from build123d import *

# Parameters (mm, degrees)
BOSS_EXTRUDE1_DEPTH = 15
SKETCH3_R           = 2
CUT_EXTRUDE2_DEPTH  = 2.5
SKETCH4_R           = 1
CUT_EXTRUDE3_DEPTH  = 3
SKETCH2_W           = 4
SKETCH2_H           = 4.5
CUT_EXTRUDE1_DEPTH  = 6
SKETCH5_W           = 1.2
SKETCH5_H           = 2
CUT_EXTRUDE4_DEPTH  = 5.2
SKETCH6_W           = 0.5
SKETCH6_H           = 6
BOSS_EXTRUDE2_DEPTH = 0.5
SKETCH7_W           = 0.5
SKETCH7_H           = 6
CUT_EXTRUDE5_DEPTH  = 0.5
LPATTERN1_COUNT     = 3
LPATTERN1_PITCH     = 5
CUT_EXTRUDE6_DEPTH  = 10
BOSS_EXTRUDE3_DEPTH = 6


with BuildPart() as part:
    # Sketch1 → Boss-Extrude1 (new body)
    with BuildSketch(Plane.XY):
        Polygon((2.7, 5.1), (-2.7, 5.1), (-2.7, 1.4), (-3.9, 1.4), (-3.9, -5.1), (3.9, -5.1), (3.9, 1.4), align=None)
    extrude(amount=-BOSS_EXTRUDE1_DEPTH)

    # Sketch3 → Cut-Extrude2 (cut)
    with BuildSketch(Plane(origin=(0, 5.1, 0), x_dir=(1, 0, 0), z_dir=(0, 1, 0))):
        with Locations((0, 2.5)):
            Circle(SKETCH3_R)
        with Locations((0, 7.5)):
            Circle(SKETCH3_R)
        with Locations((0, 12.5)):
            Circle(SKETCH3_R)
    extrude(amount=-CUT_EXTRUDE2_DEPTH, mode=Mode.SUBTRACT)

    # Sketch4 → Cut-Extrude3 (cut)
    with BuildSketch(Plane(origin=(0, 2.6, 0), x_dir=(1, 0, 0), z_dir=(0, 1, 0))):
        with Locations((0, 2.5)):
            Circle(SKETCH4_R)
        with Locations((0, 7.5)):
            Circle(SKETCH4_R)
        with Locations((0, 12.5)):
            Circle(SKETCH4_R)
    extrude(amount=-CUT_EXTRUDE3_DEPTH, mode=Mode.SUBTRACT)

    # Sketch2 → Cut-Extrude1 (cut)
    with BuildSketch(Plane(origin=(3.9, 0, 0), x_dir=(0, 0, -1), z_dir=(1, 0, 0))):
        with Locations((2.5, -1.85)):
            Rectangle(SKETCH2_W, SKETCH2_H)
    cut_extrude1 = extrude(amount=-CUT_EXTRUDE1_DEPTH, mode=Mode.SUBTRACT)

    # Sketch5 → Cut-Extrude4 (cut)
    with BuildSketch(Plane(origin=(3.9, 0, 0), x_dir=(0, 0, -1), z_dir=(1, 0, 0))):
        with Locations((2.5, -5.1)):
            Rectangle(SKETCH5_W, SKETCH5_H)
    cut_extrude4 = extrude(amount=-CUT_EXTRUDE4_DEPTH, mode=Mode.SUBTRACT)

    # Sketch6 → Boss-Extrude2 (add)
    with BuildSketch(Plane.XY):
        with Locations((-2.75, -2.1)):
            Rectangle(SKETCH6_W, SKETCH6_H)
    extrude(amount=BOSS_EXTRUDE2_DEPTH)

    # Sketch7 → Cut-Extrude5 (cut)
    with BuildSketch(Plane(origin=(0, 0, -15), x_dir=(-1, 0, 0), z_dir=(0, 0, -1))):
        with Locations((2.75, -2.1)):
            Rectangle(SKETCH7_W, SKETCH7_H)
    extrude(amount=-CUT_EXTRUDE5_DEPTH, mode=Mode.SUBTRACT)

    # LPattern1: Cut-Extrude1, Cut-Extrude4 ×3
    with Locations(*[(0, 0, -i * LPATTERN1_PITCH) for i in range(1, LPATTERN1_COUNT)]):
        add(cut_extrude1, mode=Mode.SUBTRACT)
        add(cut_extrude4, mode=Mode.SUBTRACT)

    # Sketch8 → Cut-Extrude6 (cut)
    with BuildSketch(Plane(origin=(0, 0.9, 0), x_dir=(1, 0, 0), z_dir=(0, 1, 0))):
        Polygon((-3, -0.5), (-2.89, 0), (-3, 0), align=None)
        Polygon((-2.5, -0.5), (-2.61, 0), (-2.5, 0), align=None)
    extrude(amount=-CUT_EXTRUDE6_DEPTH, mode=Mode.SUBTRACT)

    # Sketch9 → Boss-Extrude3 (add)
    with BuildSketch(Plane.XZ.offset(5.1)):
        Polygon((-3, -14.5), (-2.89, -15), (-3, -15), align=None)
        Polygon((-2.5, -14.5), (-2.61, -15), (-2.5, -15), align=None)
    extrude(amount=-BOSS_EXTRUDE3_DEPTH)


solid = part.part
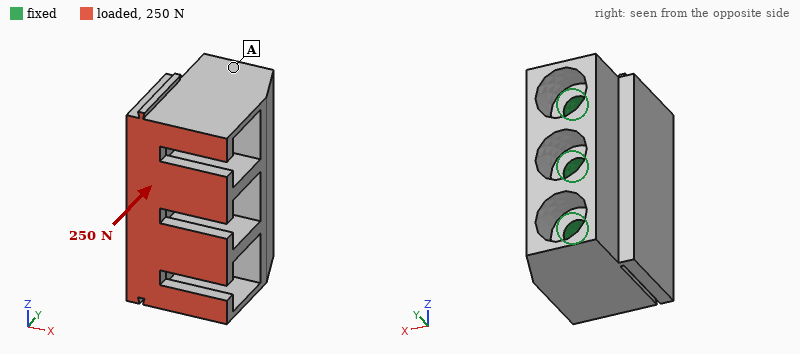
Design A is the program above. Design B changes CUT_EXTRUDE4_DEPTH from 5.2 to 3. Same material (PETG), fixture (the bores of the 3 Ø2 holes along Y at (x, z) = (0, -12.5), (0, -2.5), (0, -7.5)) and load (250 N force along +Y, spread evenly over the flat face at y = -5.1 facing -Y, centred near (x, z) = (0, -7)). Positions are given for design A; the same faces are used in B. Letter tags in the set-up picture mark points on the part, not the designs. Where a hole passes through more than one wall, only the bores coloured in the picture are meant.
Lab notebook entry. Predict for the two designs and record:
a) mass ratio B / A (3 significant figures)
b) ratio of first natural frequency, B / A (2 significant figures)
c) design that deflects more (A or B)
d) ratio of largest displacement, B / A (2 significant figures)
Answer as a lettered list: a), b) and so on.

a) 1.01
b) 1.0
c) A
d) 0.64
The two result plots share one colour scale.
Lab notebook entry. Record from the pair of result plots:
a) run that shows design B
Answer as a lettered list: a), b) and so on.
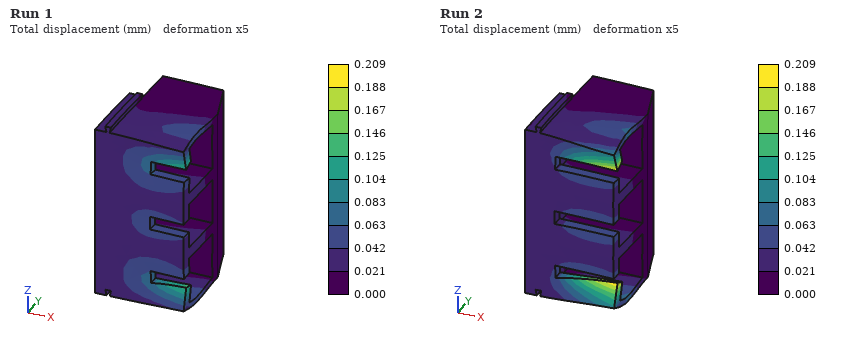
a) Run 1
